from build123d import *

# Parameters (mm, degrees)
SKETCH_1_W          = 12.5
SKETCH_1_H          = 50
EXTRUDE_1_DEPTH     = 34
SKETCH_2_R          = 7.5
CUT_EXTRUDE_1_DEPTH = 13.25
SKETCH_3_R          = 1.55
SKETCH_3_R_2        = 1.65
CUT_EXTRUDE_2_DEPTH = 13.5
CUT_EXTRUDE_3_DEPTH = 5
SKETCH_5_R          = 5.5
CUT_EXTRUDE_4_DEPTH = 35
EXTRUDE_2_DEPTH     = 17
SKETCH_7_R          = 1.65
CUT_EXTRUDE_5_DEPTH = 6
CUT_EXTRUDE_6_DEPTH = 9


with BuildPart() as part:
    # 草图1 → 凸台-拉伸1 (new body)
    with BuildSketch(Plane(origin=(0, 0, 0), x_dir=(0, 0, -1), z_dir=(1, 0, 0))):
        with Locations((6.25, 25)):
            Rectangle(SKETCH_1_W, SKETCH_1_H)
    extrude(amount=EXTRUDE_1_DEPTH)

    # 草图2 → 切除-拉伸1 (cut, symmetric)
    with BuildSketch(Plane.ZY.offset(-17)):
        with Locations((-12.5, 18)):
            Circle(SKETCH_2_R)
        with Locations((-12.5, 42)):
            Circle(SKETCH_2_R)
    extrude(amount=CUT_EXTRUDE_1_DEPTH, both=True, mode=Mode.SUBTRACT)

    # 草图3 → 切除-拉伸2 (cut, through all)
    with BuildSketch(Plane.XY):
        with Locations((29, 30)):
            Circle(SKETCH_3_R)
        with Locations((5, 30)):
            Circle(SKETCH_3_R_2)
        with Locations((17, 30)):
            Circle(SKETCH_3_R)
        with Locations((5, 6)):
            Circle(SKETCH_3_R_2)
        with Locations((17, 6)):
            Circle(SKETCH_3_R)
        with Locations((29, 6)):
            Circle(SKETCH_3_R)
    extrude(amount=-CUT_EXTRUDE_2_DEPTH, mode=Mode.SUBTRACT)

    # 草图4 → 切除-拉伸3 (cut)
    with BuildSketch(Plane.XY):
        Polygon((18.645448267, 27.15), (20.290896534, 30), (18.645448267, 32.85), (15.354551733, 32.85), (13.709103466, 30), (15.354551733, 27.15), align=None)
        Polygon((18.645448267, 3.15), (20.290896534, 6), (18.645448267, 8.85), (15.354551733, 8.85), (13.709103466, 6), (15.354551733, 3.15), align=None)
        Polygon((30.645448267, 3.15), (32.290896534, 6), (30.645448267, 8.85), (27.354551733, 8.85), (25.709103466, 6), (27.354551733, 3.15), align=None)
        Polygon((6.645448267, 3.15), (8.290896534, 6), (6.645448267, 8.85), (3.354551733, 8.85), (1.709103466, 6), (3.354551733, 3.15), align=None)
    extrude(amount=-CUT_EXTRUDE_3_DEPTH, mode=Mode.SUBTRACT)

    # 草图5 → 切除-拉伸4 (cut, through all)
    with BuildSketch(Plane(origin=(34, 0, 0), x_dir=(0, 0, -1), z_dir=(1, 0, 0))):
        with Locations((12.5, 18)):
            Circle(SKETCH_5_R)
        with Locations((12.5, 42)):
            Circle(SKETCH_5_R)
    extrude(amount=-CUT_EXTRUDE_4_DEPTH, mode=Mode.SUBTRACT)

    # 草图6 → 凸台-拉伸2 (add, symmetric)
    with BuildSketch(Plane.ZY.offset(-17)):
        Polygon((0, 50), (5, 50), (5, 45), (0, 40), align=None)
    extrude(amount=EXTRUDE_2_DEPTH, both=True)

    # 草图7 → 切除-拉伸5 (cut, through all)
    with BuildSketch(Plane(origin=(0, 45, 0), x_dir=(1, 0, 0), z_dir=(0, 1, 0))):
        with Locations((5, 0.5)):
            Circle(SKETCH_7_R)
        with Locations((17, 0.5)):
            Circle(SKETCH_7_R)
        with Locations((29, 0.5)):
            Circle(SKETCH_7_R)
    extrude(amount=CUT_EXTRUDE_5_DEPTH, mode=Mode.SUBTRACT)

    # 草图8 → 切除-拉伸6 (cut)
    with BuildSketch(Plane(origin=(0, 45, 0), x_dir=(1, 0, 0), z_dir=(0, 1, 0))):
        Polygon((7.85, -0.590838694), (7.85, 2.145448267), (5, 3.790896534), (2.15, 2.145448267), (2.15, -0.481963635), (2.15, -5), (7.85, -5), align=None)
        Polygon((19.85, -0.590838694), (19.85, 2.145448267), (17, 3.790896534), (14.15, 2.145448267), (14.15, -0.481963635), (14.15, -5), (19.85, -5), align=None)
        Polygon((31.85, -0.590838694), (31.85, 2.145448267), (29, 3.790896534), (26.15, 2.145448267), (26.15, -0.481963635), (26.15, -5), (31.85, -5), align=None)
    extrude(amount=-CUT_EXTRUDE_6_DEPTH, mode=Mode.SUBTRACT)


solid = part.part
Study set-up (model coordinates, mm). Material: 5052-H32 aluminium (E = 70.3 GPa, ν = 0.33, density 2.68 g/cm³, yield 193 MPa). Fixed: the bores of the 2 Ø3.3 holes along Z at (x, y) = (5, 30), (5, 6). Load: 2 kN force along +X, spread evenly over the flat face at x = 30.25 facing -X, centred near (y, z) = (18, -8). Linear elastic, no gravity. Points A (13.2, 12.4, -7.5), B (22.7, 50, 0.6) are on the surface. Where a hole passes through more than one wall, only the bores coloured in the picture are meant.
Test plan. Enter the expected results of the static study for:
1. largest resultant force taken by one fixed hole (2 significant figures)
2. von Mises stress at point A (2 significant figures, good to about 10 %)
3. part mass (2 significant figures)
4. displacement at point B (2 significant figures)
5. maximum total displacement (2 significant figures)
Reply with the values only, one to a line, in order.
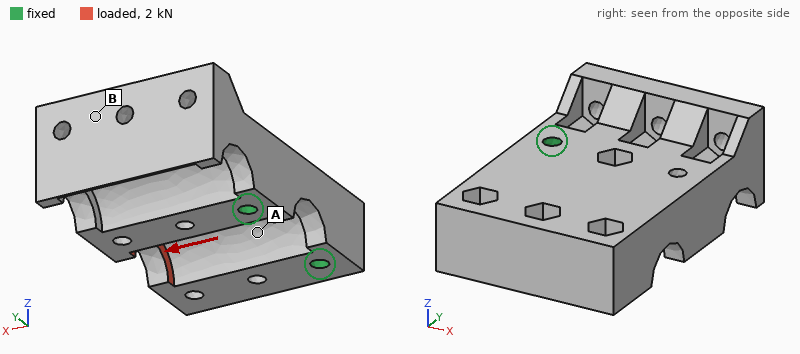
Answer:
1.0 kN
11 MPa
41 g
3.5 µm
16 µm
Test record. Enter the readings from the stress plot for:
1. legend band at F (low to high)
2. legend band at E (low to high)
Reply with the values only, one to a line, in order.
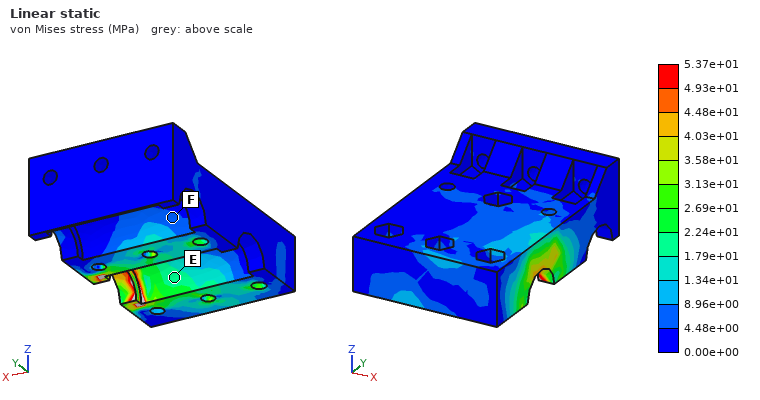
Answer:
4.48e+00 to 8.96e+00 MPa
1.79e+01 to 2.24e+01 MPa
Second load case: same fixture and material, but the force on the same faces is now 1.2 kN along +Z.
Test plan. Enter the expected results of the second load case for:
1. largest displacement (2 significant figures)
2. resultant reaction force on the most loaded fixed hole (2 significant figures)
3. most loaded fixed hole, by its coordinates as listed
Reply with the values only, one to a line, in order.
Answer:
58 µm
740 N
(5, 30)
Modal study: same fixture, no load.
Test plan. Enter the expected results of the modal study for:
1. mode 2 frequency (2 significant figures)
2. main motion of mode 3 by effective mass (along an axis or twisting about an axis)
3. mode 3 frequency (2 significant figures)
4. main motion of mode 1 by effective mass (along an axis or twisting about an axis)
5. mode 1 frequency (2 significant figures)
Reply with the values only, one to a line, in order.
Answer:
8200 Hz
along Y
11 kHz
along Z
6700 Hz
